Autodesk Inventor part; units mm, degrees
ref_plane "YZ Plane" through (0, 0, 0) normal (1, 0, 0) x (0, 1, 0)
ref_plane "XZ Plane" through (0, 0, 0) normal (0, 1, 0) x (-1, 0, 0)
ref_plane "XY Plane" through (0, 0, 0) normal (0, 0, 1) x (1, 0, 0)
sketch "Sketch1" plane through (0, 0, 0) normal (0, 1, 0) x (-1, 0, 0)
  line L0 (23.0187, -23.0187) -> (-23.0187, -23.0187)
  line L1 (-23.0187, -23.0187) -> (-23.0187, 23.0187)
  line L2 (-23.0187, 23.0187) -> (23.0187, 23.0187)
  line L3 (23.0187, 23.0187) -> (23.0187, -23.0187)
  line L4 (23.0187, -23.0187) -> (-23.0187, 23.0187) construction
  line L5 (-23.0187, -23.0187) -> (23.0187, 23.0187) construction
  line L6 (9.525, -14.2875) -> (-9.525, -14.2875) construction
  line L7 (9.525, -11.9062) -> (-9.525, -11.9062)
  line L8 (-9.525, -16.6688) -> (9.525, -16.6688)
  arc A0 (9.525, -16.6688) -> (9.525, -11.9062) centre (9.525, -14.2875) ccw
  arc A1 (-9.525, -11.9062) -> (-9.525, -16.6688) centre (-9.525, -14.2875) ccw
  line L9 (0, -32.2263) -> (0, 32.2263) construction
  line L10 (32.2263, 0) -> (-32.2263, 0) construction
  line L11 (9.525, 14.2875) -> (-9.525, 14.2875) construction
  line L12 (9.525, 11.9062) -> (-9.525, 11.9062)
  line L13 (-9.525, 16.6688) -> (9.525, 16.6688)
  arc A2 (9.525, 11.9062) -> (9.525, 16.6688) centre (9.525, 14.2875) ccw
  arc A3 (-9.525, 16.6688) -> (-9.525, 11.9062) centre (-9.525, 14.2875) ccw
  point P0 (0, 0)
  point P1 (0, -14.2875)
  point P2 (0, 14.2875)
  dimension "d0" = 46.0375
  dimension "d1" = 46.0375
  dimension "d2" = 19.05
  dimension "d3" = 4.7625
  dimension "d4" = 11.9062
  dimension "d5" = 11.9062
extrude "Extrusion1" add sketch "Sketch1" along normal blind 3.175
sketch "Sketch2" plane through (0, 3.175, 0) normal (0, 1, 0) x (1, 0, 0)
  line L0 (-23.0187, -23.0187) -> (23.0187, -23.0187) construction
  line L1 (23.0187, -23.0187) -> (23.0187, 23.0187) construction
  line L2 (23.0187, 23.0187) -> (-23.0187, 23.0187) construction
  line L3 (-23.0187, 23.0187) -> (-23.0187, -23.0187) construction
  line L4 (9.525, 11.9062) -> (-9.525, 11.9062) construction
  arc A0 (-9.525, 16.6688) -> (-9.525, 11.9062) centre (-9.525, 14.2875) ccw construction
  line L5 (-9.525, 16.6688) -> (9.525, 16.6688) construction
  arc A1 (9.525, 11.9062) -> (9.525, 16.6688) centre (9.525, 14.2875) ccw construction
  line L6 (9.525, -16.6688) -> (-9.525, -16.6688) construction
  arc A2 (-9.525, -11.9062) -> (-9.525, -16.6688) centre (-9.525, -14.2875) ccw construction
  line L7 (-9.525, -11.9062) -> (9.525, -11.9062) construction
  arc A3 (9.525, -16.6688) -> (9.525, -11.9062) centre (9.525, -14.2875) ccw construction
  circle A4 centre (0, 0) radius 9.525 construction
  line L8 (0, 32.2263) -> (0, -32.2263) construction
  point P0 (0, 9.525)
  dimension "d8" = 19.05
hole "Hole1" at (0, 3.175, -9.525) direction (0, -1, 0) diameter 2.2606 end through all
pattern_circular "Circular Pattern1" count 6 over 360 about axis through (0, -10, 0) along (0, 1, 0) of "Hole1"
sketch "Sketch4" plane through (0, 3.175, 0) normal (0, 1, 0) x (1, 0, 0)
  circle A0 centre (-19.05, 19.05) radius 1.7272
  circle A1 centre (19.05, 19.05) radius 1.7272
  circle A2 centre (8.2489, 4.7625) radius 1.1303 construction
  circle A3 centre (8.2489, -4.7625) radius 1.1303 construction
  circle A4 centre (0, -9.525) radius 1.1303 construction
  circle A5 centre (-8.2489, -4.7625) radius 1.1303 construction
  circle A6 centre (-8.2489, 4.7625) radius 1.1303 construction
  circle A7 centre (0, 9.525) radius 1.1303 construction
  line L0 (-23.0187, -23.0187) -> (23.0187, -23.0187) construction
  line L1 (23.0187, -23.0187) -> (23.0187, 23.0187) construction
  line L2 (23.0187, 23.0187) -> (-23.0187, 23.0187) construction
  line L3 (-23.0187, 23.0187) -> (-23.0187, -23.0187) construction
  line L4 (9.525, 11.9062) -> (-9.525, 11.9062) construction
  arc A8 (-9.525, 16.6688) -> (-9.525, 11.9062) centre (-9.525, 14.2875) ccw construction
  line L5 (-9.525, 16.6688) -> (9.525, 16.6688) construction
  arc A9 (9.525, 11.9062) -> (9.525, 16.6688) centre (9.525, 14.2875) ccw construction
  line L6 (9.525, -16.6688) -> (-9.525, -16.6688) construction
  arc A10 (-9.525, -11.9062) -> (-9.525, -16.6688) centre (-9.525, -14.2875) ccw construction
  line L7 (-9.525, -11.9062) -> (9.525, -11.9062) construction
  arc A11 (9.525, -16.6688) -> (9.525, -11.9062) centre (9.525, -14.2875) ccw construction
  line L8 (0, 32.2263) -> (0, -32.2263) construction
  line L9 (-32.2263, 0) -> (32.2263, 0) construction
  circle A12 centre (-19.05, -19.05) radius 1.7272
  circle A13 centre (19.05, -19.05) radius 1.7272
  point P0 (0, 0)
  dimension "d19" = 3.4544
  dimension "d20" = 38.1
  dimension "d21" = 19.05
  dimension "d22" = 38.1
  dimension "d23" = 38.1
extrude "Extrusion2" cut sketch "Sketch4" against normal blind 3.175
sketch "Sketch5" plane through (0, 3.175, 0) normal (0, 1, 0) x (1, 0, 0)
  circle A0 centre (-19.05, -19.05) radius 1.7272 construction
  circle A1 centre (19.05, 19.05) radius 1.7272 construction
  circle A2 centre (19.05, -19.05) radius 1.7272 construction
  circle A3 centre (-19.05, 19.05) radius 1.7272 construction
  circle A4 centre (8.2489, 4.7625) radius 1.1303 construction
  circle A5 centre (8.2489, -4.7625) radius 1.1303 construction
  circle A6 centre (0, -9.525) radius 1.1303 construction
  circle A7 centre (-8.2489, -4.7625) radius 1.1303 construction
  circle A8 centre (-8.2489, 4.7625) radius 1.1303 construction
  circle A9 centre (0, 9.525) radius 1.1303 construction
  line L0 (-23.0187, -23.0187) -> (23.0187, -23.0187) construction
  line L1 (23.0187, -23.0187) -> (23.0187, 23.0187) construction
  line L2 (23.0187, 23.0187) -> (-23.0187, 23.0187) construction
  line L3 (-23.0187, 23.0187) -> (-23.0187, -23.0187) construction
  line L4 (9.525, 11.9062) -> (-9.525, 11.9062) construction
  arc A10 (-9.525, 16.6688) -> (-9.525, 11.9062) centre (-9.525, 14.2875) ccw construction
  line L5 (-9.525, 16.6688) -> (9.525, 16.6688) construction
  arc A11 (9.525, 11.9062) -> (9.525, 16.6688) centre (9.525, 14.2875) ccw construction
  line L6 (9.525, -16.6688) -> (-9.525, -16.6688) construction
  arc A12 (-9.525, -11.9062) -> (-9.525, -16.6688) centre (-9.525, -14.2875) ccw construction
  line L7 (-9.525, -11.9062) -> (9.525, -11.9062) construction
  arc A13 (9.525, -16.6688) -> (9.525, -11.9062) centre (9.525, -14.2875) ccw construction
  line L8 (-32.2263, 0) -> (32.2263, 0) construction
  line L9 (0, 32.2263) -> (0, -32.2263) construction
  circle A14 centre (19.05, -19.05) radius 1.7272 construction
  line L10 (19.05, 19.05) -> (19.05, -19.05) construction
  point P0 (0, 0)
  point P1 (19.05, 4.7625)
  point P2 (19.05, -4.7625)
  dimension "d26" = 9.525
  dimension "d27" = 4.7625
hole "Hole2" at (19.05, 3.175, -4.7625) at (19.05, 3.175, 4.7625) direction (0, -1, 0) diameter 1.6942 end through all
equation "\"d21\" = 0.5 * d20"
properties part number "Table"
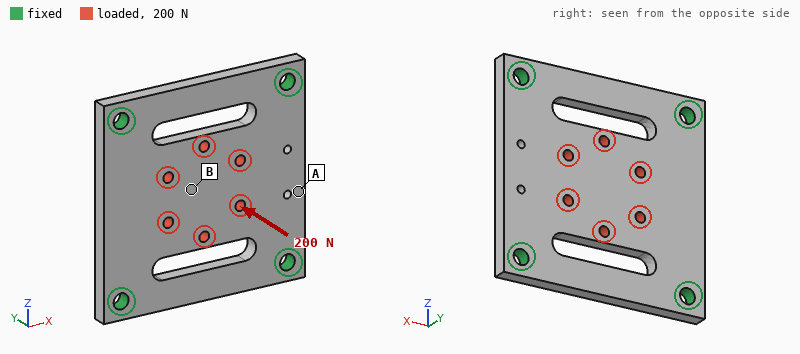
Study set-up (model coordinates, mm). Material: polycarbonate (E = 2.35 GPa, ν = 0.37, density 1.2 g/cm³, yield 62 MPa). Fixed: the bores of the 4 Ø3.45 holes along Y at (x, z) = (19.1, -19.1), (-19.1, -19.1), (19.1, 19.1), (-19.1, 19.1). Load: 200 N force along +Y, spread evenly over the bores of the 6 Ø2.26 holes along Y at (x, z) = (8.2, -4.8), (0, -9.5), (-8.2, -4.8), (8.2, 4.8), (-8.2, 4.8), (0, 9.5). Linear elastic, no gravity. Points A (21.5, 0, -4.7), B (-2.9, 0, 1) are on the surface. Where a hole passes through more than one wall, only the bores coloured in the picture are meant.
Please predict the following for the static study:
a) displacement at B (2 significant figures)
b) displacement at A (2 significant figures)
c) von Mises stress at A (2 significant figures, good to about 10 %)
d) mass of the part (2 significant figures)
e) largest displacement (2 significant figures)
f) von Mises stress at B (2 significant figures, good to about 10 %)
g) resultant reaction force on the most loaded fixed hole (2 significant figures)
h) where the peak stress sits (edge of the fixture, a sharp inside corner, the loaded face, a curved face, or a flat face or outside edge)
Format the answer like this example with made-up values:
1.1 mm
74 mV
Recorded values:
0.57 mm
0.10 mm
5.3 MPa
7.0 g
0.58 mm
12 MPa
50 N
the loaded face
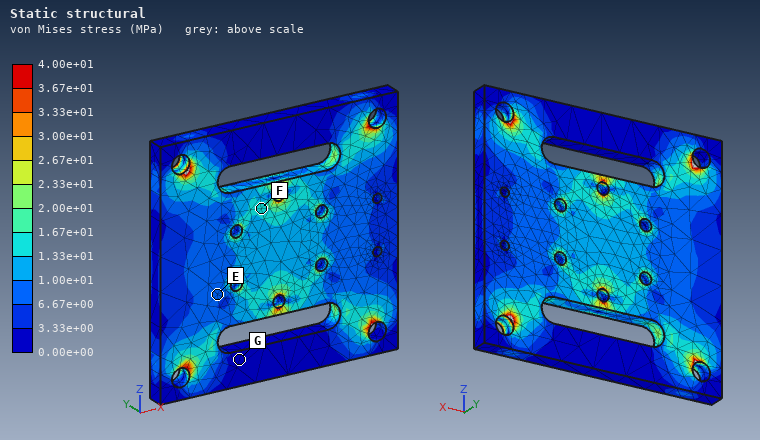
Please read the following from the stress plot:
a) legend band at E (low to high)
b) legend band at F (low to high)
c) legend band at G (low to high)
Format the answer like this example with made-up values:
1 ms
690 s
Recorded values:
6.67e+00 to 1.00e+01 MPa
1.33e+01 to 1.67e+01 MPa
0.00e+00 to 3.33e+00 MPa
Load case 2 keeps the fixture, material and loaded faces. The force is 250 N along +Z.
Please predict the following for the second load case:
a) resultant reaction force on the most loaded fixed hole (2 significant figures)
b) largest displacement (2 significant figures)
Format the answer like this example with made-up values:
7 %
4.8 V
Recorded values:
69 N
37 µm
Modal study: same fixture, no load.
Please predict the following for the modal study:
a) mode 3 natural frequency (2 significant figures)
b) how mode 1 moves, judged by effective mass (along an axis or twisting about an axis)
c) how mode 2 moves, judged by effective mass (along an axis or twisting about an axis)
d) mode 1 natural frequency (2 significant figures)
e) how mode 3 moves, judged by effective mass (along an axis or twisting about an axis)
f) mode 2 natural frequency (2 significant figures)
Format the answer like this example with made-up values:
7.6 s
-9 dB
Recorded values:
3700 Hz
along Y
twisting about Z
2000 Hz
twisting about X
3400 Hz
